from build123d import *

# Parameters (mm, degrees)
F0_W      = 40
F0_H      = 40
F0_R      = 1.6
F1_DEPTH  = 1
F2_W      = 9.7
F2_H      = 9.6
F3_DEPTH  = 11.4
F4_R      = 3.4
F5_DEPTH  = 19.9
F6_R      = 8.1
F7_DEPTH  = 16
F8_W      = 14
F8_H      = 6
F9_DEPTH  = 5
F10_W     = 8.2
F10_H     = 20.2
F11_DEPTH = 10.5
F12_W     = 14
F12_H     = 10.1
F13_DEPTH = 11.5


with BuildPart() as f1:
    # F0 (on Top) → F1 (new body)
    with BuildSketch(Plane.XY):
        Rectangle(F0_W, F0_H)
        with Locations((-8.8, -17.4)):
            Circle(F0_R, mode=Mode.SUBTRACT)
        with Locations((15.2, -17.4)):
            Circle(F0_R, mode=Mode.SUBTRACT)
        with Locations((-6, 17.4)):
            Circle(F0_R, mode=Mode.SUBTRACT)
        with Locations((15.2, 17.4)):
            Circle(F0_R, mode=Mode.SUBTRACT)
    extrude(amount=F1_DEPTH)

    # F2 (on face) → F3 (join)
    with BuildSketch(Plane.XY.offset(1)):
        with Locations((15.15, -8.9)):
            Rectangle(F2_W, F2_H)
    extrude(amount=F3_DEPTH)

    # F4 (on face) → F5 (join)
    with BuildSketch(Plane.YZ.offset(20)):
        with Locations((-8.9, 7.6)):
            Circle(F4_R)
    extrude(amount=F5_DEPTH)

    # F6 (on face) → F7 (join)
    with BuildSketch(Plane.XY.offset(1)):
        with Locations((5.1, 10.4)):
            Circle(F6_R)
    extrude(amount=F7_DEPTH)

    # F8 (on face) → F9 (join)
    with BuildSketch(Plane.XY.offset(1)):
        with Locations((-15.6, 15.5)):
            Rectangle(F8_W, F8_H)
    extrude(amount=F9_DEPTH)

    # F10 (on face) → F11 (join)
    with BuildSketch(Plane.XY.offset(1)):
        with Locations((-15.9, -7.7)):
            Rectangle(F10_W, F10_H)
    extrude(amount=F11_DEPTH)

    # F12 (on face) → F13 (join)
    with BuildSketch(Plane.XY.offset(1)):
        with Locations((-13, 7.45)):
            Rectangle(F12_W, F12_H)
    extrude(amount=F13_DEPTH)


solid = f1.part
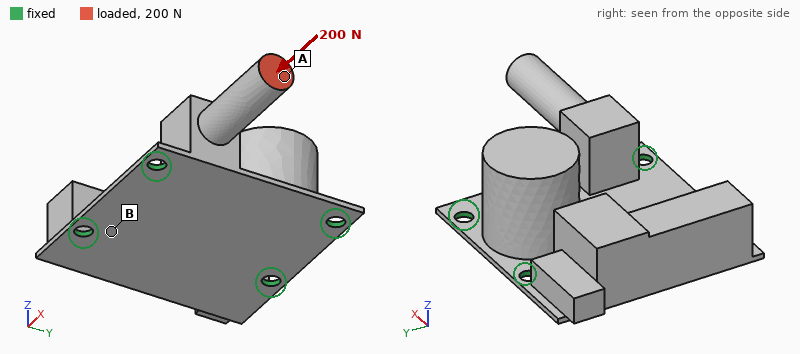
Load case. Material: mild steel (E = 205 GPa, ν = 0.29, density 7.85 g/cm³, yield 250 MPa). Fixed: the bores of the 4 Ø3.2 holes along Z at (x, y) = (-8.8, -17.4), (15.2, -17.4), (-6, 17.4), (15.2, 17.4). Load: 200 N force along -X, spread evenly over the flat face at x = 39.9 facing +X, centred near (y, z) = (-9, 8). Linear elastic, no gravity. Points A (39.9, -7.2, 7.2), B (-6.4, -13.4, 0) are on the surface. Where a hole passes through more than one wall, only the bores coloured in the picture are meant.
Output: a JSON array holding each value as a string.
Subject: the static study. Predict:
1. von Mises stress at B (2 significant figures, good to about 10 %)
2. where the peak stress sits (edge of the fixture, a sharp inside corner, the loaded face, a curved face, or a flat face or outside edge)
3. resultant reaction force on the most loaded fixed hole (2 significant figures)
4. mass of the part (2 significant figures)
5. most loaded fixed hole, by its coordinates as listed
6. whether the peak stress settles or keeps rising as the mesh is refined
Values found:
["33 MPa", "edge of the fixture", "100 N", "82 g", "(15.2, -17.4)", "keeps rising"]
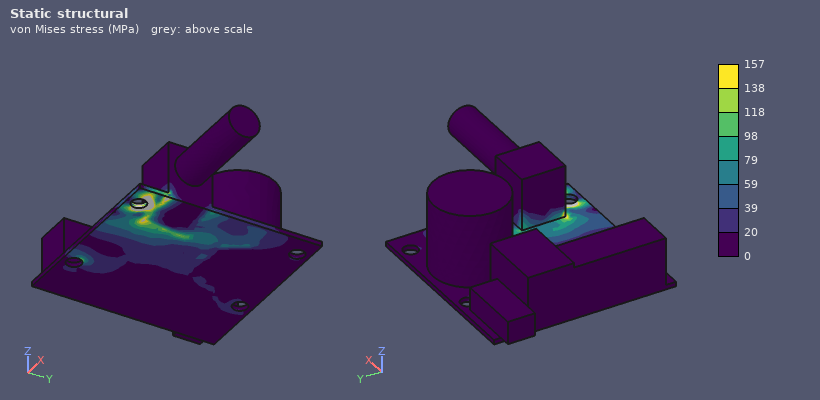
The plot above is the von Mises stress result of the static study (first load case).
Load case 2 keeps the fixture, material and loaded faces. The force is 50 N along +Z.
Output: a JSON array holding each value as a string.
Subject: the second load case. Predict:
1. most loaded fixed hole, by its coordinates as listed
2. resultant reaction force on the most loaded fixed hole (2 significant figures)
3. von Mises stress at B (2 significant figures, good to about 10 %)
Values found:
["(15.2, -17.4)", "65 N", "25 MPa"]
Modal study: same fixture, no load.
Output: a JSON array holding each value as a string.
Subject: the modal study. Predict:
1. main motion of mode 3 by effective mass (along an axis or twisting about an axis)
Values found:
["along Z"]
